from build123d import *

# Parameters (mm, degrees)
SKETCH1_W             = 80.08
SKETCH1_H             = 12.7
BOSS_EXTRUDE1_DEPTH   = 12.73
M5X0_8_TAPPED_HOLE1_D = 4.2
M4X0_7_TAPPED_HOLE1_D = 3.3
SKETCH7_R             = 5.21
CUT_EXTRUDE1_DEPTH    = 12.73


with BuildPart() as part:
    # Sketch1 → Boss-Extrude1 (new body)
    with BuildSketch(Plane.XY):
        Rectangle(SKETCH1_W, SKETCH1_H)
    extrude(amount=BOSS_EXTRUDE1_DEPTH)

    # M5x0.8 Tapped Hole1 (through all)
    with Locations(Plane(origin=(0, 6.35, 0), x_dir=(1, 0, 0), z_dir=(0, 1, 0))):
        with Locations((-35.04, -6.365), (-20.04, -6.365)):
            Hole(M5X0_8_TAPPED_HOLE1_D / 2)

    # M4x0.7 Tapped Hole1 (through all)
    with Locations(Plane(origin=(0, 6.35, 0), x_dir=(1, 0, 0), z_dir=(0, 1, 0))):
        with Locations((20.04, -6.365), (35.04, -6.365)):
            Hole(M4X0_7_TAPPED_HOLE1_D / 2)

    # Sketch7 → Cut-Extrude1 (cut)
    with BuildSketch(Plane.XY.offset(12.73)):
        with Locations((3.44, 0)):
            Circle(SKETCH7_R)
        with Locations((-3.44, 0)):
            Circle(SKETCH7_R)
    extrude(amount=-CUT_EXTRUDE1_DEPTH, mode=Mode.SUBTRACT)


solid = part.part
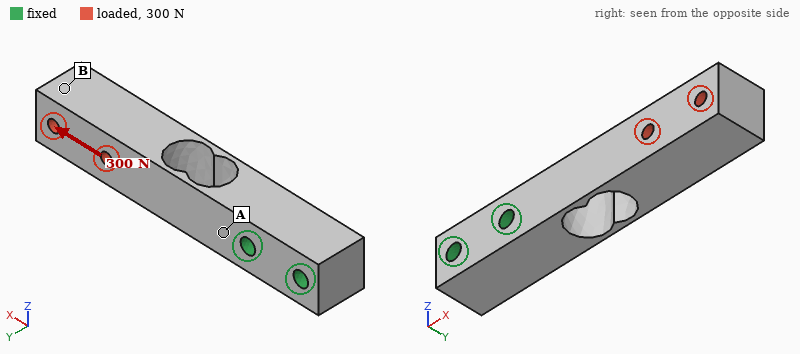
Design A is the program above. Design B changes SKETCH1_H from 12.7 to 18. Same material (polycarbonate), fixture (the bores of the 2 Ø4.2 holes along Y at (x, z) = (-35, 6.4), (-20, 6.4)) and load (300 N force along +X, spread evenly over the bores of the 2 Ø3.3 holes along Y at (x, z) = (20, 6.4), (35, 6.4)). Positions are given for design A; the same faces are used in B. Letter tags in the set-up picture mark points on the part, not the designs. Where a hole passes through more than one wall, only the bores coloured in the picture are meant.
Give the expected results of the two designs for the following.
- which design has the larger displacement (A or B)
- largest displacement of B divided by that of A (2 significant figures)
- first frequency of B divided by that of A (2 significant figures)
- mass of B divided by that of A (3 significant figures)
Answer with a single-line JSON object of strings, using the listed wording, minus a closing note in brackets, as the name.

{"which design has the larger displacement": "A", "largest displacement of B divided by that of A": "0.44", "first frequency of B divided by that of A": "1.5", "mass of B divided by that of A": "1.49"}
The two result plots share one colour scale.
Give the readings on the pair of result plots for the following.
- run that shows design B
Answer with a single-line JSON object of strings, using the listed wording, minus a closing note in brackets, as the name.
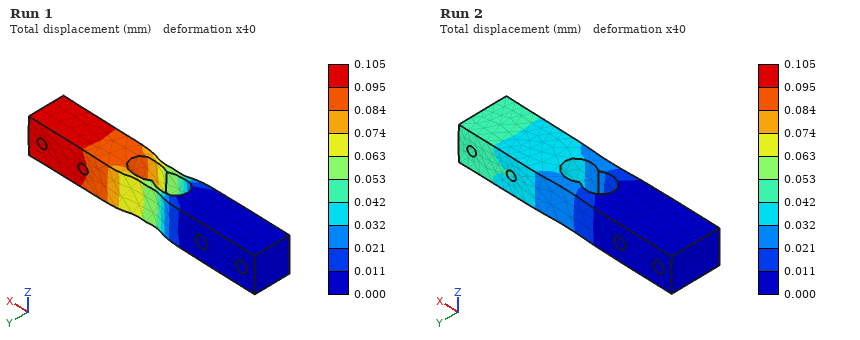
{"run that shows design B": "Run 2"}
